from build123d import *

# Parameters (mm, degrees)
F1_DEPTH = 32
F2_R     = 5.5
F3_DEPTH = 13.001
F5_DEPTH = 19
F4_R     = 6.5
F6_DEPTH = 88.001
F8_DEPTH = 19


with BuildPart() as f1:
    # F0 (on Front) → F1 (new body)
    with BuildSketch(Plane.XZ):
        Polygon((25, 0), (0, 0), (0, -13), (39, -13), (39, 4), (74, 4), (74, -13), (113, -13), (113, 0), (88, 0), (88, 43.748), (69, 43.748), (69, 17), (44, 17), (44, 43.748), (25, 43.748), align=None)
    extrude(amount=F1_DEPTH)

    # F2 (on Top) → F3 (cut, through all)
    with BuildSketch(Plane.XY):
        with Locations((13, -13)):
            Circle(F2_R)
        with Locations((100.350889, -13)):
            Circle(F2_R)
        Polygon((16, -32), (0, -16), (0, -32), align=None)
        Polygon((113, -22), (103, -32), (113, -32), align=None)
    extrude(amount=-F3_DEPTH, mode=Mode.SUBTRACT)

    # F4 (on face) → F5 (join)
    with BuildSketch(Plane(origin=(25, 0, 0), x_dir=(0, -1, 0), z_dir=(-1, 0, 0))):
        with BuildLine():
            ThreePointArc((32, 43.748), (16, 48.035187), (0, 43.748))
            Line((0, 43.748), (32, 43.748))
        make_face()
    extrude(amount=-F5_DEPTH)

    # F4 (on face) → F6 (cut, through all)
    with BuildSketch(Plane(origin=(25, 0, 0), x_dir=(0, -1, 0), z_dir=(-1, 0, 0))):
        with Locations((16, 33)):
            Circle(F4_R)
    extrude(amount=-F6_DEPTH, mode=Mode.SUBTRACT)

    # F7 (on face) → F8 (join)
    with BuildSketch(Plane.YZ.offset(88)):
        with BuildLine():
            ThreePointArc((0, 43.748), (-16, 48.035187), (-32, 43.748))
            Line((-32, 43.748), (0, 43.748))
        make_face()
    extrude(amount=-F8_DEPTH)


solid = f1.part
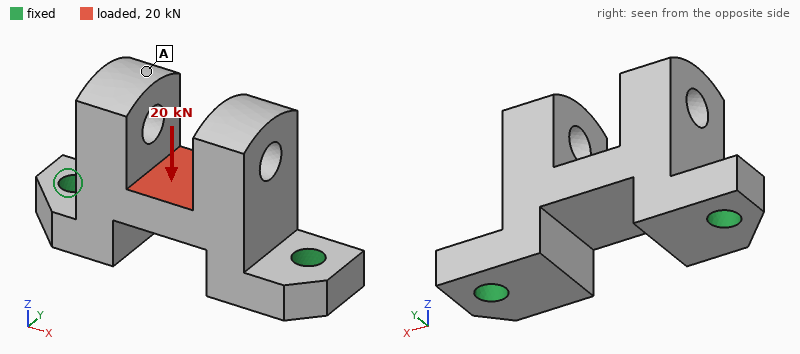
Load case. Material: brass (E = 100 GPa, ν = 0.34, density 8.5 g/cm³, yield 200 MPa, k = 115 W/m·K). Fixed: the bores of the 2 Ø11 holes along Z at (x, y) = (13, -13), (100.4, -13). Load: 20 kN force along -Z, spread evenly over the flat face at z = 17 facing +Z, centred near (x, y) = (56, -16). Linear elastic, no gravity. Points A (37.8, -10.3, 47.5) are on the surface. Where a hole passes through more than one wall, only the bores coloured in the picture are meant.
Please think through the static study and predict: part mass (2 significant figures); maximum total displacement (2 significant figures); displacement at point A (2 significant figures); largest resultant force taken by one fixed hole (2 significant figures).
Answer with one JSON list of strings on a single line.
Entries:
["750 g", "68 µm", "62 µm", "15 kN"]
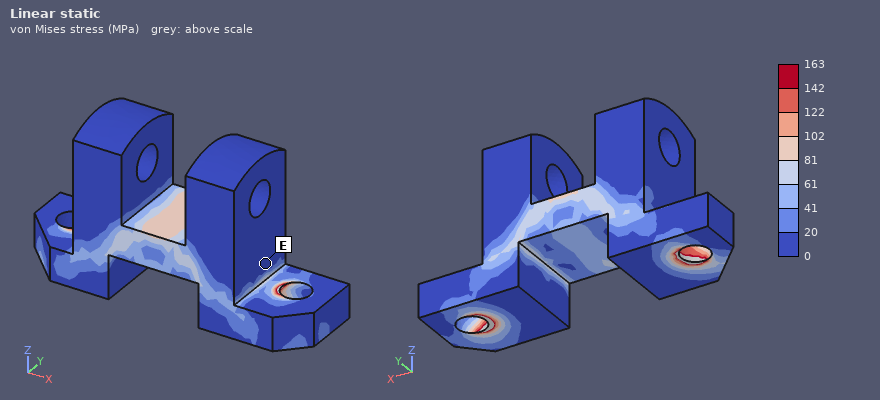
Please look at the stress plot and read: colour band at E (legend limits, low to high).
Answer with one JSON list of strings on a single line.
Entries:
["0 to 20 MPa"]
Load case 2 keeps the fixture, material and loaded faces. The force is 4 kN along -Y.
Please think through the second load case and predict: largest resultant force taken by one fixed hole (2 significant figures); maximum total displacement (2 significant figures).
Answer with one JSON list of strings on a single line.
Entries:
["2.0 kN", "58 µm"]
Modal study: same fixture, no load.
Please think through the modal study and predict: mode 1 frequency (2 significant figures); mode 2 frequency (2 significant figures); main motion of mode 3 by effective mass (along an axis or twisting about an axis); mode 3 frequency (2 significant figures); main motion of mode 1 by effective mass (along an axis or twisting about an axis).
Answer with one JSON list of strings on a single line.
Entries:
["2000 Hz", "3400 Hz", "along X", "4300 Hz", "along Y"]
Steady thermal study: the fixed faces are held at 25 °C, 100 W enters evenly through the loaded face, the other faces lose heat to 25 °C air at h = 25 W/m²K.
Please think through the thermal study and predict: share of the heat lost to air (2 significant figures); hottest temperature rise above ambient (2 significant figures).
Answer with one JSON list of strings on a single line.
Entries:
["9.7 %", "43 K"]
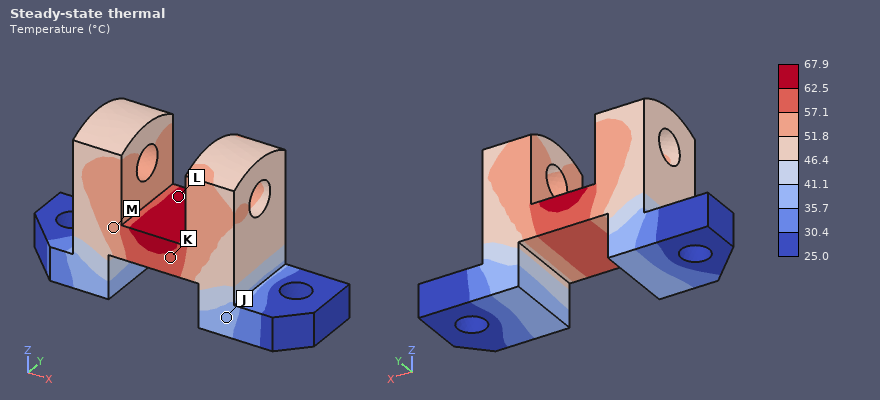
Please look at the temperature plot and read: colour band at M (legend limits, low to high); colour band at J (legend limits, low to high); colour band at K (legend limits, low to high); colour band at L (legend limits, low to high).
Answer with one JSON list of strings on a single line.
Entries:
["51.8 to 57.1 °C", "35.7 to 41.1 °C", "57.1 to 62.5 °C", "62.5 to 67.9 °C"]
